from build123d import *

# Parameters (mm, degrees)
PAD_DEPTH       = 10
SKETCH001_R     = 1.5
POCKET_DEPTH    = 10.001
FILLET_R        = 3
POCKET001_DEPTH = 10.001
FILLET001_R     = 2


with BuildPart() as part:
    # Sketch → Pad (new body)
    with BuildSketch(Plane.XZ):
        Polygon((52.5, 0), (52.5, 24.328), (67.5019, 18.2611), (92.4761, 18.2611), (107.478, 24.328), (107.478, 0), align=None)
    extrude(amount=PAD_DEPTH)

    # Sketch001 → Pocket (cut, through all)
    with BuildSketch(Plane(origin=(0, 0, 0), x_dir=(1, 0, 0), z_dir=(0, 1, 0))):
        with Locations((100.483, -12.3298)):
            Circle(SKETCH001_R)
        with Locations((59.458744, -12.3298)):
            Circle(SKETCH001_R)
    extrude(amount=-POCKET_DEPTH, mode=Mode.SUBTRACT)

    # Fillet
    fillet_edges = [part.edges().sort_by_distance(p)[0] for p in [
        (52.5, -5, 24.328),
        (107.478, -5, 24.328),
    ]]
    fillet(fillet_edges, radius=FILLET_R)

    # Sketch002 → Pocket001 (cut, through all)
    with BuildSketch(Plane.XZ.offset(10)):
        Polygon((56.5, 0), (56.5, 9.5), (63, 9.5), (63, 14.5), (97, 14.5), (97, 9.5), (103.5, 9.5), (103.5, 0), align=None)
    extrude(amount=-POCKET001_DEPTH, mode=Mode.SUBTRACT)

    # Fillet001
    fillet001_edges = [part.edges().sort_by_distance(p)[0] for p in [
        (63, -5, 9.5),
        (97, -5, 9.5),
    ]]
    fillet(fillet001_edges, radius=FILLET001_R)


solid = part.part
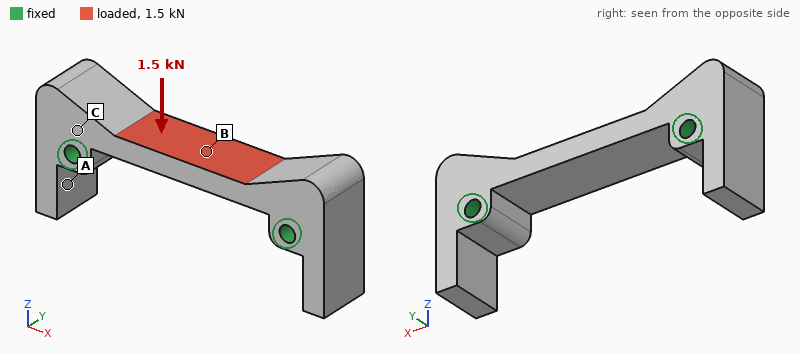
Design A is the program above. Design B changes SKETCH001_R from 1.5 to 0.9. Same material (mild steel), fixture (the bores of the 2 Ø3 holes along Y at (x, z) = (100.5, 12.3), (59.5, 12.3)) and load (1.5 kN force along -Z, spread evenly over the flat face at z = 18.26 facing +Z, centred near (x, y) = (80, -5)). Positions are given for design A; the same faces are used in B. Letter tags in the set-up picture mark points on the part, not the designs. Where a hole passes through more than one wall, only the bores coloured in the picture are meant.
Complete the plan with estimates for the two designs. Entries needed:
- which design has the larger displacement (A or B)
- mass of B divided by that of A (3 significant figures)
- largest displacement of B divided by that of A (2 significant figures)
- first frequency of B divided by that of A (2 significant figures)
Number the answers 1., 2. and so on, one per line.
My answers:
1. B
2. 1.02
3. 1.1
4. 0.90
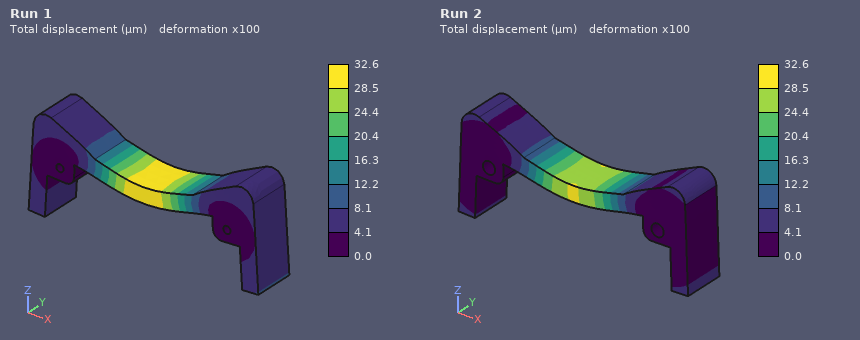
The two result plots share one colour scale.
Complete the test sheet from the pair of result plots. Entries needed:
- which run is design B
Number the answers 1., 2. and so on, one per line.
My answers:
1. Run 1
